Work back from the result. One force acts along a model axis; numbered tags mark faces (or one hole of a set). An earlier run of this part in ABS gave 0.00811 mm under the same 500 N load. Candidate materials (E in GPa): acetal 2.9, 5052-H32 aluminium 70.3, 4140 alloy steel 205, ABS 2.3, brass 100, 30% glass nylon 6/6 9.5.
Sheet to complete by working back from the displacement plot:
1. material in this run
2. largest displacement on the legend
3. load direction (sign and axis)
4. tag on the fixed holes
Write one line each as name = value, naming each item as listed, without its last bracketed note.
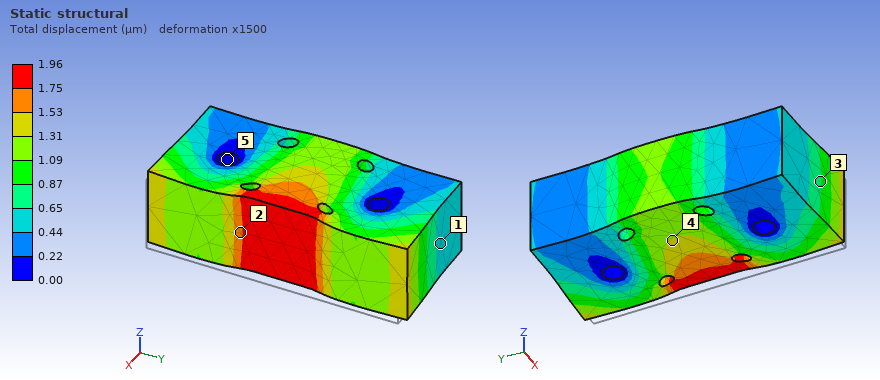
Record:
material in this run = 30% glass nylon 6/6
largest displacement on the legend = 1.96 µm
load direction = -X
tag on the fixed holes = 5
